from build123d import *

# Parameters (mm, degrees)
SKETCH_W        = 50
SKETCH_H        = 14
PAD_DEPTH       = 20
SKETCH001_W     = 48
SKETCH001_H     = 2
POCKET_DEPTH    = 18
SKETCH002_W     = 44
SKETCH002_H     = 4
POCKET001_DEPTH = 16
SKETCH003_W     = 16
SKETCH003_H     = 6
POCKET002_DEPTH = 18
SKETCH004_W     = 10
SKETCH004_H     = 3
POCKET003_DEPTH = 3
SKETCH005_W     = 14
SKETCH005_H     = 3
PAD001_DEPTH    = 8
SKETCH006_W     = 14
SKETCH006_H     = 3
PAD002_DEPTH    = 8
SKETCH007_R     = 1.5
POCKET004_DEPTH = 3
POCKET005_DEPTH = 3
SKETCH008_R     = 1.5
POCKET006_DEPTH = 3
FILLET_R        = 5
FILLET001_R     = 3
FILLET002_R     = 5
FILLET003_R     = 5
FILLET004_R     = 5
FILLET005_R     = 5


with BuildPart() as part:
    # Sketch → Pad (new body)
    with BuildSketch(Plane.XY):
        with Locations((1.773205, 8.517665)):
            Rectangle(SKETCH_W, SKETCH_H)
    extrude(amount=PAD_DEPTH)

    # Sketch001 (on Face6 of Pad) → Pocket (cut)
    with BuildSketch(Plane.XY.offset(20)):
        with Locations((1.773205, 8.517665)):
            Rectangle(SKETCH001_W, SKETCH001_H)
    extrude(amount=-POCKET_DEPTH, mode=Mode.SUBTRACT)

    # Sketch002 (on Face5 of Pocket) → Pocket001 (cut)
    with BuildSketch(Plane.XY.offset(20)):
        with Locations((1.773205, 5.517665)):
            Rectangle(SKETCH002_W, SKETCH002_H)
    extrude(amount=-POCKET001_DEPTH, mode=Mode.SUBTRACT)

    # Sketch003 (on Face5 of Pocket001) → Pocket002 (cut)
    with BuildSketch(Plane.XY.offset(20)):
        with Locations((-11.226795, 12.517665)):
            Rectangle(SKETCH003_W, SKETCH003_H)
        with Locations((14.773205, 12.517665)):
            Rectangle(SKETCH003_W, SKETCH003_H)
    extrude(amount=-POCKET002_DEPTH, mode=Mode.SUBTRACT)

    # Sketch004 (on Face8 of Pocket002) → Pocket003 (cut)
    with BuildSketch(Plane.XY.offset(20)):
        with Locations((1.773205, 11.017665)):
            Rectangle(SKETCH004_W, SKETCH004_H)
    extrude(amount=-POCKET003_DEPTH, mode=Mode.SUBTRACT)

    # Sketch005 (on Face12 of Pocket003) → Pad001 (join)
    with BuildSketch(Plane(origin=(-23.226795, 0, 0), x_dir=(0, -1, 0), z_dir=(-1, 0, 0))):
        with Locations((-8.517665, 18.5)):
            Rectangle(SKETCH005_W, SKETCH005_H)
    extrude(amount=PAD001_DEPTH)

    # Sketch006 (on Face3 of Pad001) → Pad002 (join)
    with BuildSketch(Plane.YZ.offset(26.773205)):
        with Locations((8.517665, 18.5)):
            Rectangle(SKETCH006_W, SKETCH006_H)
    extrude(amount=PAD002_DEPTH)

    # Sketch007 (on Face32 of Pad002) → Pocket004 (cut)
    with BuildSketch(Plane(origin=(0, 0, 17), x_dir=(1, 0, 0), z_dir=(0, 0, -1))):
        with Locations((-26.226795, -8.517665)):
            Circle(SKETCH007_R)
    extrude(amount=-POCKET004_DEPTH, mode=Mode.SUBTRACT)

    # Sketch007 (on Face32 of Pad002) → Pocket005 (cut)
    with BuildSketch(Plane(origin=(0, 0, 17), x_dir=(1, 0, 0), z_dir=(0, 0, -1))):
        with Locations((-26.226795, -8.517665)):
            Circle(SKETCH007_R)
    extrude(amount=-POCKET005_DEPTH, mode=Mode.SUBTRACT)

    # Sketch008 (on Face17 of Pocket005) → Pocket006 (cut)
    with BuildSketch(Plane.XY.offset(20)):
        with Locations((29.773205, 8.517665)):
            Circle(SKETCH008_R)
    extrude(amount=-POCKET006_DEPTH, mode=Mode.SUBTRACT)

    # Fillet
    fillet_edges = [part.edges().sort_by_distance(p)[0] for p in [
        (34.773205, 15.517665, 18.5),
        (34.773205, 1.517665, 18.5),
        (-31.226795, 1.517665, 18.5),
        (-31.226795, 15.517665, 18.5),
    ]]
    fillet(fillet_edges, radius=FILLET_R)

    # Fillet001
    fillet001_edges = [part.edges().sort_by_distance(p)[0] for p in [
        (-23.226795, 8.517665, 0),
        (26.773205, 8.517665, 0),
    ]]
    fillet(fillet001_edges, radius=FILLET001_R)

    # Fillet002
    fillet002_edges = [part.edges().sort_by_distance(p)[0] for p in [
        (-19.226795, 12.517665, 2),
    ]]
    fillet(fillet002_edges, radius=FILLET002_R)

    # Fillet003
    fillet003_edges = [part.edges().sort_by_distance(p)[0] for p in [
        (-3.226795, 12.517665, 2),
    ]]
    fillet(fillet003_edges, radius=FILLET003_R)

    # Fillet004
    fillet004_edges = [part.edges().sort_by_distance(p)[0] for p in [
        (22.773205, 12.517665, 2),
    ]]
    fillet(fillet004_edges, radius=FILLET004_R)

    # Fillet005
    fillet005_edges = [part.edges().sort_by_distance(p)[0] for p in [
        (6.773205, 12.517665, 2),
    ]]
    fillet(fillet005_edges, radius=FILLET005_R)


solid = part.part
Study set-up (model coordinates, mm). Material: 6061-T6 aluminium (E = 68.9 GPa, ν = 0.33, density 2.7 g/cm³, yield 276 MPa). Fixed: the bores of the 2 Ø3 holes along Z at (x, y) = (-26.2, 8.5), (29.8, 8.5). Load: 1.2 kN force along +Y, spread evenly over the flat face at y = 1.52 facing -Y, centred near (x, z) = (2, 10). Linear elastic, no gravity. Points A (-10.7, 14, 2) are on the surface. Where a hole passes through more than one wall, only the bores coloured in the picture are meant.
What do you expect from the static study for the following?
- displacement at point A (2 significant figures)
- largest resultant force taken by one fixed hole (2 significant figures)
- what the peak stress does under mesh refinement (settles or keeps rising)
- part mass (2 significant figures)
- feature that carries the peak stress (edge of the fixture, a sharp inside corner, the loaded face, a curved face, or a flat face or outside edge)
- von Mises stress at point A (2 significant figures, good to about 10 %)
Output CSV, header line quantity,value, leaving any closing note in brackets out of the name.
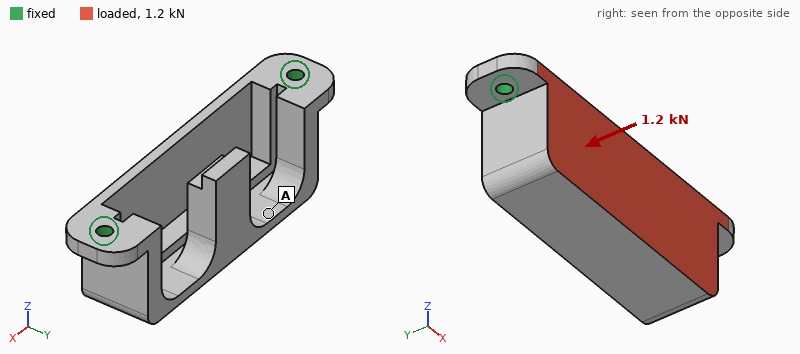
quantity,value
displacement at point A,0.12 mm
largest resultant force taken by one fixed hole,660 N
what the peak stress does under mesh refinement,keeps rising
part mass,18 g
feature that carries the peak stress,edge of the fixture
von Mises stress at point A,44 MPa
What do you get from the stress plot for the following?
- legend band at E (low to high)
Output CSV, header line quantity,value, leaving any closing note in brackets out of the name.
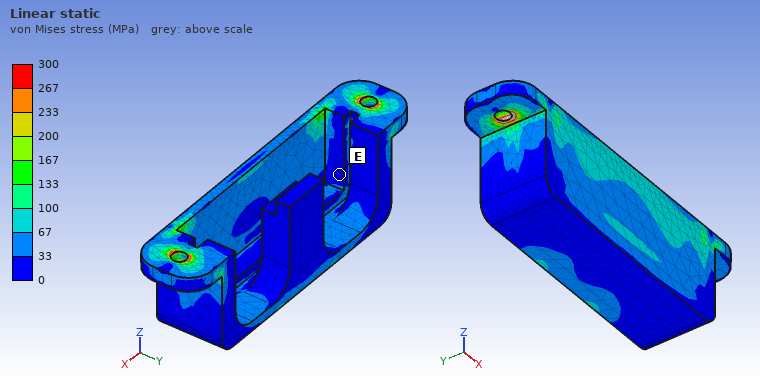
quantity,value
legend band at E,0 to 33 MPa
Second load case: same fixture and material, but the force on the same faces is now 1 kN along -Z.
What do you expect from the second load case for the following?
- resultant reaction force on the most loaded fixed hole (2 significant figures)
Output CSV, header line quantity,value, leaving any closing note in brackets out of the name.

quantity,value
resultant reaction force on the most loaded fixed hole,560 N
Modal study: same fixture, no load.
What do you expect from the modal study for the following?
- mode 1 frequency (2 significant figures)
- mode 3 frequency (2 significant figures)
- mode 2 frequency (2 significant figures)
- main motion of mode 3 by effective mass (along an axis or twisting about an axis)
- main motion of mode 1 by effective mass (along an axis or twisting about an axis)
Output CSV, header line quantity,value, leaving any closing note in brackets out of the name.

quantity,value
mode 1 frequency,3600 Hz
mode 3 frequency,5200 Hz
mode 2 frequency,4300 Hz
main motion of mode 3 by effective mass,along X
main motion of mode 1 by effective mass,along Y
